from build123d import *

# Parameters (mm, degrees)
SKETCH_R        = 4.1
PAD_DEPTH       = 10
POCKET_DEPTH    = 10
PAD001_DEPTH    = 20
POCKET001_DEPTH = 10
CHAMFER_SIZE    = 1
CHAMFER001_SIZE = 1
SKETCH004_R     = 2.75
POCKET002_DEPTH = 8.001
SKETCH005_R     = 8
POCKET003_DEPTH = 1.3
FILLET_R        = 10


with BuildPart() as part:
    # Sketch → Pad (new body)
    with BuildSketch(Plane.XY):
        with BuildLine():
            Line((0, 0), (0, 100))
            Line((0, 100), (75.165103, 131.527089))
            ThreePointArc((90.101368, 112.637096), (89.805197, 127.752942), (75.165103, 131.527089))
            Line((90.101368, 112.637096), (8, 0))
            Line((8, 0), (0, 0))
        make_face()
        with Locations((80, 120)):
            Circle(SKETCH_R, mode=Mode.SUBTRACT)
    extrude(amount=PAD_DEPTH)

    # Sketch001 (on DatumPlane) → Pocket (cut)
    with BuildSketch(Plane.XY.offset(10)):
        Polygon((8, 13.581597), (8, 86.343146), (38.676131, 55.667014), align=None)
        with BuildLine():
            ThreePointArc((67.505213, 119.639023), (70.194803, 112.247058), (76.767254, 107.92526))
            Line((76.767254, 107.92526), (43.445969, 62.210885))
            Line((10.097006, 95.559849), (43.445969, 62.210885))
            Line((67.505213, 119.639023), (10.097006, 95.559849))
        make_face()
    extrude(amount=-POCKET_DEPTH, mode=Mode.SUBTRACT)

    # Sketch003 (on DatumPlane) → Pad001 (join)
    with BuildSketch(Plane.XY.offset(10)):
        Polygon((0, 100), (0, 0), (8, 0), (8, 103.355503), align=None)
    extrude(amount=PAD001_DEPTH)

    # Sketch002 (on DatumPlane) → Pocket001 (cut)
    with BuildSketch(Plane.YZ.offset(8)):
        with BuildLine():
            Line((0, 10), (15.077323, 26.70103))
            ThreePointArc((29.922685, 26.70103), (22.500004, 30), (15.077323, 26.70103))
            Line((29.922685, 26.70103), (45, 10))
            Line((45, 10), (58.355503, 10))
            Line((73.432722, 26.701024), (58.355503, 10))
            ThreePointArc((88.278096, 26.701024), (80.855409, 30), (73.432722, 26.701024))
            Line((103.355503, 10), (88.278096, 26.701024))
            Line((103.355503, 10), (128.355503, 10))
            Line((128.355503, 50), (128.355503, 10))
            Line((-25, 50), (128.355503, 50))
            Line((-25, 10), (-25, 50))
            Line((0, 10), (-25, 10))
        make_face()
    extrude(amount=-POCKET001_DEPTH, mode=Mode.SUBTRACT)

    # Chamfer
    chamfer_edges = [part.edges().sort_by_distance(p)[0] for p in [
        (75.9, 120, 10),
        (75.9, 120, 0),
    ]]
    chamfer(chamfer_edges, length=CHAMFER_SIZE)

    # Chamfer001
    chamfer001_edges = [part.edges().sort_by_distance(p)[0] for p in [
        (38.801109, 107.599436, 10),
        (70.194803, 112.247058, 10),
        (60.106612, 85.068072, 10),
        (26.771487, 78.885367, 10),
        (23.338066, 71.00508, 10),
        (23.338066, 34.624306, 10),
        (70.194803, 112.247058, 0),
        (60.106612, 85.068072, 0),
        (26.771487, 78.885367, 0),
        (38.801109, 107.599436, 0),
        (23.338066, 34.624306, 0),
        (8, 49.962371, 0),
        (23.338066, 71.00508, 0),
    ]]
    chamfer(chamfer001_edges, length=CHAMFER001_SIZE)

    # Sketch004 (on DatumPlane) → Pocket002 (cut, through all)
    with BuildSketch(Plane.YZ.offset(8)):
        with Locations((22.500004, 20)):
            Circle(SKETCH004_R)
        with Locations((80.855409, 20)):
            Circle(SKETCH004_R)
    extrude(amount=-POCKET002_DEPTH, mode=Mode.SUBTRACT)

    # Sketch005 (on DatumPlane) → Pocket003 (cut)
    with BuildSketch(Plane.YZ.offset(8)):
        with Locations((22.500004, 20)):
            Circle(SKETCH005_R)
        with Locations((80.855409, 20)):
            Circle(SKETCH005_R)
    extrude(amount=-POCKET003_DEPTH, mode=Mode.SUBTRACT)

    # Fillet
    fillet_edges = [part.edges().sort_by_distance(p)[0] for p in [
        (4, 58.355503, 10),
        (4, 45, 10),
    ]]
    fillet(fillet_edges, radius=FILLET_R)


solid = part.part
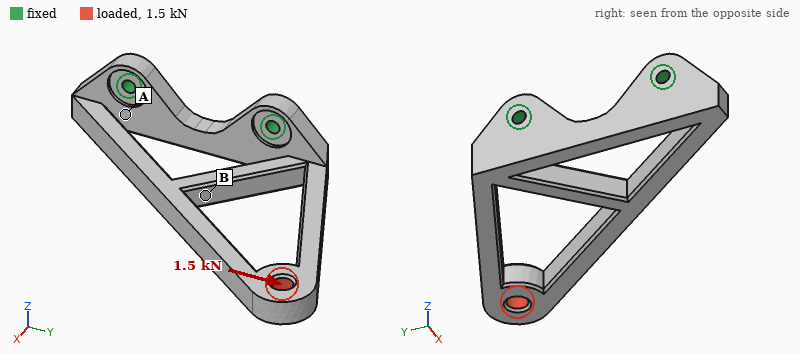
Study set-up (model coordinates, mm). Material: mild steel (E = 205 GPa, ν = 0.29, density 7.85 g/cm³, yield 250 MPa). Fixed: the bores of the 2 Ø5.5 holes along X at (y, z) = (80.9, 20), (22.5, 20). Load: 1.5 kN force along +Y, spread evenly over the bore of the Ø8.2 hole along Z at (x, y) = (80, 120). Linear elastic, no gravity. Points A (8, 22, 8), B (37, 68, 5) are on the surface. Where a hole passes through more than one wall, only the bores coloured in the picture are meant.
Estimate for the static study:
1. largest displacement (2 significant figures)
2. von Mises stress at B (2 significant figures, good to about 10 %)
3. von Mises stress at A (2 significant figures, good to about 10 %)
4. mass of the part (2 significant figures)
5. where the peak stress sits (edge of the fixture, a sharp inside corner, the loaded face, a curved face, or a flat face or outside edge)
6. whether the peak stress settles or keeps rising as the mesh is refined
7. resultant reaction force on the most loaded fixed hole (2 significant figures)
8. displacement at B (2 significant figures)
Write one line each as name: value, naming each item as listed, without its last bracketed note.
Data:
largest displacement: 0.14 mm
von Mises stress at B: 21 MPa
von Mises stress at A: 66 MPa
mass of the part: 310 g
where the peak stress sits: edge of the fixture
whether the peak stress settles or keeps rising as the mesh is refined: keeps rising
resultant reaction force on the most loaded fixed hole: 1.8 kN
displacement at B: 0.029 mm
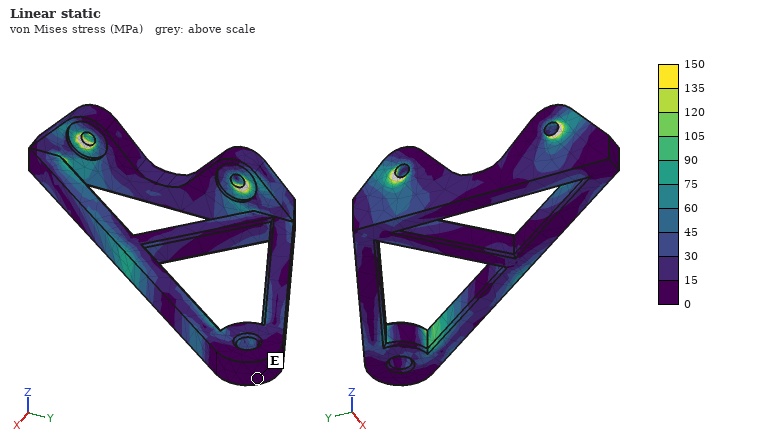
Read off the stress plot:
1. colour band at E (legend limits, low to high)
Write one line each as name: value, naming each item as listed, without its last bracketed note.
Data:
colour band at E: 0 to 15 MPa
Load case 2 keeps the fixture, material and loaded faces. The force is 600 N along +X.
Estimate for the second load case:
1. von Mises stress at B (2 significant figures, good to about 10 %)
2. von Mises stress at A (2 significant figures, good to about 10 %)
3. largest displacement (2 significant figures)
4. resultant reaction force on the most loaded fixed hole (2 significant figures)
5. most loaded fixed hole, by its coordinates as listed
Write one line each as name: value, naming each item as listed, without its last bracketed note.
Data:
von Mises stress at B: 9.9 MPa
von Mises stress at A: 10 MPa
largest displacement: 64 µm
resultant reaction force on the most loaded fixed hole: 840 N
most loaded fixed hole, by its coordinates as listed: (80.9, 20)
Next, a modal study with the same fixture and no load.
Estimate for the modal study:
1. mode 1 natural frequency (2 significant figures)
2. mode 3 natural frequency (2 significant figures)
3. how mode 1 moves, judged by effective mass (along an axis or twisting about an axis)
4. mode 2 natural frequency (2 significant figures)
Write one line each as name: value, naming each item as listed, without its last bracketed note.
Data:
mode 1 natural frequency: 600 Hz
mode 3 natural frequency: 2100 Hz
how mode 1 moves, judged by effective mass: along Z
mode 2 natural frequency: 1700 Hz
